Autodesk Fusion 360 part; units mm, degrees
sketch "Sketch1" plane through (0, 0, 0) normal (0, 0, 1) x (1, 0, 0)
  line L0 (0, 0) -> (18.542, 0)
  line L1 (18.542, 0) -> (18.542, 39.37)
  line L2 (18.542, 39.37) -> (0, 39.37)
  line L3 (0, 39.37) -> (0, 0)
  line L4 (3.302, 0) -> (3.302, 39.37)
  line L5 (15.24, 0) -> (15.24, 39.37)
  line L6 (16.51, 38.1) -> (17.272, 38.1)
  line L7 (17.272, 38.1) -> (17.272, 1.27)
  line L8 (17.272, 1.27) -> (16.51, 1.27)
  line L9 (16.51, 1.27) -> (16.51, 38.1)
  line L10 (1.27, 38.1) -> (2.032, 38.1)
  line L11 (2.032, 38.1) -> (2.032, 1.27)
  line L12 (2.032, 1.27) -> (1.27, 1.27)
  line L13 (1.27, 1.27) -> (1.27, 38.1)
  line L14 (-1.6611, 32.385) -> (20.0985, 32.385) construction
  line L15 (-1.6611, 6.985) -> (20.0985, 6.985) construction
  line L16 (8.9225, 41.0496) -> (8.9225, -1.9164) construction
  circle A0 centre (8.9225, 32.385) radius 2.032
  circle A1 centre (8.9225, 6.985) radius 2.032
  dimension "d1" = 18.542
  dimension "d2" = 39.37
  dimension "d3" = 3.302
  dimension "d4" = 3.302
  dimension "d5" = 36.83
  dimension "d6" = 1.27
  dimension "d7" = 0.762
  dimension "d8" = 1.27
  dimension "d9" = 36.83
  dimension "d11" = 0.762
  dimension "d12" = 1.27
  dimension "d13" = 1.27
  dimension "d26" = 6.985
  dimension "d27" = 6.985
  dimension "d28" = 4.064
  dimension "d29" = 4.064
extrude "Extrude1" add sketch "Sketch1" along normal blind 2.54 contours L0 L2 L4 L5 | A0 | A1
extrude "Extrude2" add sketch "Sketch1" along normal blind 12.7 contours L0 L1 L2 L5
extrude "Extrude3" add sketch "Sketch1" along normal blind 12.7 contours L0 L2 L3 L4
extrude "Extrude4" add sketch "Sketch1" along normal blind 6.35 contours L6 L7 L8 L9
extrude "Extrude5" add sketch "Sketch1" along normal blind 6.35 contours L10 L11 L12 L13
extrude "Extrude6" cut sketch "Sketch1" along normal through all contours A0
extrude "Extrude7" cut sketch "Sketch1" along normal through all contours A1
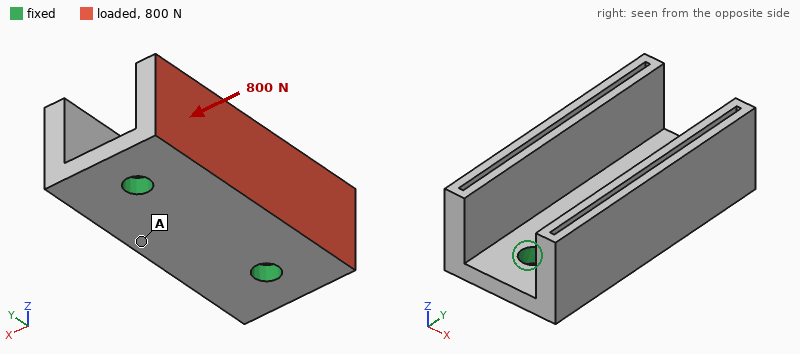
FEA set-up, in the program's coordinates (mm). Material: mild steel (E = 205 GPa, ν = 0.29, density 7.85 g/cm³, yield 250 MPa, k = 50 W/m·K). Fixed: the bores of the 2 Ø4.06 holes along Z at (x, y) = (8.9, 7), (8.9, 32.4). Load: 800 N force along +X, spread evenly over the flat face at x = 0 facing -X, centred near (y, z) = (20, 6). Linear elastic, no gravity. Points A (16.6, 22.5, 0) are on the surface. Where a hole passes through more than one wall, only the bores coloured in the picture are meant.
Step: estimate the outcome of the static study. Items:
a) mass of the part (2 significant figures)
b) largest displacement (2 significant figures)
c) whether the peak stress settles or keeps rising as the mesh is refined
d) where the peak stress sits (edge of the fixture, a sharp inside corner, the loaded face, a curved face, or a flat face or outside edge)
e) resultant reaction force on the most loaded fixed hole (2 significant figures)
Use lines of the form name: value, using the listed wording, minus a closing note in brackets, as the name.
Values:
mass of the part: 32 g
largest displacement: 43 µm
whether the peak stress settles or keeps rising as the mesh is refined: keeps rising
where the peak stress sits: edge of the fixture
resultant reaction force on the most loaded fixed hole: 400 N
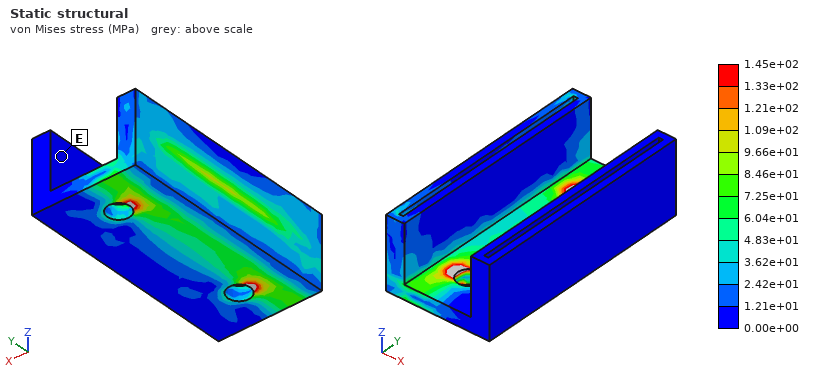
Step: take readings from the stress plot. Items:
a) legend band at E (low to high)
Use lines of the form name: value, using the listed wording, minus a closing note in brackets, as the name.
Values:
legend band at E: 0.00e+00 to 1.21e+01 MPa
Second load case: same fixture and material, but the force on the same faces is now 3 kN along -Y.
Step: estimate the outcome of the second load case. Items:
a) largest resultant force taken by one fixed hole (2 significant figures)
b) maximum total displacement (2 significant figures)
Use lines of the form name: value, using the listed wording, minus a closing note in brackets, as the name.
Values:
largest resultant force taken by one fixed hole: 1.8 kN
maximum total displacement: 22 µm
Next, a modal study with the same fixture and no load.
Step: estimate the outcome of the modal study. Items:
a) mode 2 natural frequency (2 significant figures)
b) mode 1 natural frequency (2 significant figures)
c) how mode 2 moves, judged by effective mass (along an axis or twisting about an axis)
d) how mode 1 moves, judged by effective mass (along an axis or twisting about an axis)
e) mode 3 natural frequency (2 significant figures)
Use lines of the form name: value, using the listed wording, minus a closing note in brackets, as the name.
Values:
mode 2 natural frequency: 8400 Hz
mode 1 natural frequency: 7400 Hz
how mode 2 moves, judged by effective mass: along Z
how mode 1 moves, judged by effective mass: along X
mode 3 natural frequency: 11 kHz
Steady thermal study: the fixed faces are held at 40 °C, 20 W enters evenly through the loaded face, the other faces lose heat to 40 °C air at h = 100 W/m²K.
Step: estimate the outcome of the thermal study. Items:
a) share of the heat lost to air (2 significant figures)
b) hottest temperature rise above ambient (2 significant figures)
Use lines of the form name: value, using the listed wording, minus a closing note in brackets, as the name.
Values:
share of the heat lost to air: 27 %
hottest temperature rise above ambient: 46 K
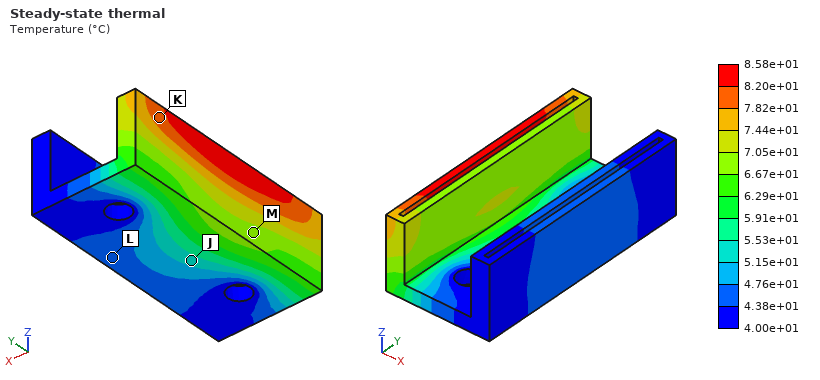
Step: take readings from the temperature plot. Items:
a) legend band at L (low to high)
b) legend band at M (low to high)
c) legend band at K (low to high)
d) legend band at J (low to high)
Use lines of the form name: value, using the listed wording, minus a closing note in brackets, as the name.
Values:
legend band at L: 4.38e+01 to 4.76e+01 °C
legend band at M: 6.67e+01 to 7.05e+01 °C
legend band at K: 7.82e+01 to 8.20e+01 °C
legend band at J: 5.15e+01 to 5.53e+01 °C
